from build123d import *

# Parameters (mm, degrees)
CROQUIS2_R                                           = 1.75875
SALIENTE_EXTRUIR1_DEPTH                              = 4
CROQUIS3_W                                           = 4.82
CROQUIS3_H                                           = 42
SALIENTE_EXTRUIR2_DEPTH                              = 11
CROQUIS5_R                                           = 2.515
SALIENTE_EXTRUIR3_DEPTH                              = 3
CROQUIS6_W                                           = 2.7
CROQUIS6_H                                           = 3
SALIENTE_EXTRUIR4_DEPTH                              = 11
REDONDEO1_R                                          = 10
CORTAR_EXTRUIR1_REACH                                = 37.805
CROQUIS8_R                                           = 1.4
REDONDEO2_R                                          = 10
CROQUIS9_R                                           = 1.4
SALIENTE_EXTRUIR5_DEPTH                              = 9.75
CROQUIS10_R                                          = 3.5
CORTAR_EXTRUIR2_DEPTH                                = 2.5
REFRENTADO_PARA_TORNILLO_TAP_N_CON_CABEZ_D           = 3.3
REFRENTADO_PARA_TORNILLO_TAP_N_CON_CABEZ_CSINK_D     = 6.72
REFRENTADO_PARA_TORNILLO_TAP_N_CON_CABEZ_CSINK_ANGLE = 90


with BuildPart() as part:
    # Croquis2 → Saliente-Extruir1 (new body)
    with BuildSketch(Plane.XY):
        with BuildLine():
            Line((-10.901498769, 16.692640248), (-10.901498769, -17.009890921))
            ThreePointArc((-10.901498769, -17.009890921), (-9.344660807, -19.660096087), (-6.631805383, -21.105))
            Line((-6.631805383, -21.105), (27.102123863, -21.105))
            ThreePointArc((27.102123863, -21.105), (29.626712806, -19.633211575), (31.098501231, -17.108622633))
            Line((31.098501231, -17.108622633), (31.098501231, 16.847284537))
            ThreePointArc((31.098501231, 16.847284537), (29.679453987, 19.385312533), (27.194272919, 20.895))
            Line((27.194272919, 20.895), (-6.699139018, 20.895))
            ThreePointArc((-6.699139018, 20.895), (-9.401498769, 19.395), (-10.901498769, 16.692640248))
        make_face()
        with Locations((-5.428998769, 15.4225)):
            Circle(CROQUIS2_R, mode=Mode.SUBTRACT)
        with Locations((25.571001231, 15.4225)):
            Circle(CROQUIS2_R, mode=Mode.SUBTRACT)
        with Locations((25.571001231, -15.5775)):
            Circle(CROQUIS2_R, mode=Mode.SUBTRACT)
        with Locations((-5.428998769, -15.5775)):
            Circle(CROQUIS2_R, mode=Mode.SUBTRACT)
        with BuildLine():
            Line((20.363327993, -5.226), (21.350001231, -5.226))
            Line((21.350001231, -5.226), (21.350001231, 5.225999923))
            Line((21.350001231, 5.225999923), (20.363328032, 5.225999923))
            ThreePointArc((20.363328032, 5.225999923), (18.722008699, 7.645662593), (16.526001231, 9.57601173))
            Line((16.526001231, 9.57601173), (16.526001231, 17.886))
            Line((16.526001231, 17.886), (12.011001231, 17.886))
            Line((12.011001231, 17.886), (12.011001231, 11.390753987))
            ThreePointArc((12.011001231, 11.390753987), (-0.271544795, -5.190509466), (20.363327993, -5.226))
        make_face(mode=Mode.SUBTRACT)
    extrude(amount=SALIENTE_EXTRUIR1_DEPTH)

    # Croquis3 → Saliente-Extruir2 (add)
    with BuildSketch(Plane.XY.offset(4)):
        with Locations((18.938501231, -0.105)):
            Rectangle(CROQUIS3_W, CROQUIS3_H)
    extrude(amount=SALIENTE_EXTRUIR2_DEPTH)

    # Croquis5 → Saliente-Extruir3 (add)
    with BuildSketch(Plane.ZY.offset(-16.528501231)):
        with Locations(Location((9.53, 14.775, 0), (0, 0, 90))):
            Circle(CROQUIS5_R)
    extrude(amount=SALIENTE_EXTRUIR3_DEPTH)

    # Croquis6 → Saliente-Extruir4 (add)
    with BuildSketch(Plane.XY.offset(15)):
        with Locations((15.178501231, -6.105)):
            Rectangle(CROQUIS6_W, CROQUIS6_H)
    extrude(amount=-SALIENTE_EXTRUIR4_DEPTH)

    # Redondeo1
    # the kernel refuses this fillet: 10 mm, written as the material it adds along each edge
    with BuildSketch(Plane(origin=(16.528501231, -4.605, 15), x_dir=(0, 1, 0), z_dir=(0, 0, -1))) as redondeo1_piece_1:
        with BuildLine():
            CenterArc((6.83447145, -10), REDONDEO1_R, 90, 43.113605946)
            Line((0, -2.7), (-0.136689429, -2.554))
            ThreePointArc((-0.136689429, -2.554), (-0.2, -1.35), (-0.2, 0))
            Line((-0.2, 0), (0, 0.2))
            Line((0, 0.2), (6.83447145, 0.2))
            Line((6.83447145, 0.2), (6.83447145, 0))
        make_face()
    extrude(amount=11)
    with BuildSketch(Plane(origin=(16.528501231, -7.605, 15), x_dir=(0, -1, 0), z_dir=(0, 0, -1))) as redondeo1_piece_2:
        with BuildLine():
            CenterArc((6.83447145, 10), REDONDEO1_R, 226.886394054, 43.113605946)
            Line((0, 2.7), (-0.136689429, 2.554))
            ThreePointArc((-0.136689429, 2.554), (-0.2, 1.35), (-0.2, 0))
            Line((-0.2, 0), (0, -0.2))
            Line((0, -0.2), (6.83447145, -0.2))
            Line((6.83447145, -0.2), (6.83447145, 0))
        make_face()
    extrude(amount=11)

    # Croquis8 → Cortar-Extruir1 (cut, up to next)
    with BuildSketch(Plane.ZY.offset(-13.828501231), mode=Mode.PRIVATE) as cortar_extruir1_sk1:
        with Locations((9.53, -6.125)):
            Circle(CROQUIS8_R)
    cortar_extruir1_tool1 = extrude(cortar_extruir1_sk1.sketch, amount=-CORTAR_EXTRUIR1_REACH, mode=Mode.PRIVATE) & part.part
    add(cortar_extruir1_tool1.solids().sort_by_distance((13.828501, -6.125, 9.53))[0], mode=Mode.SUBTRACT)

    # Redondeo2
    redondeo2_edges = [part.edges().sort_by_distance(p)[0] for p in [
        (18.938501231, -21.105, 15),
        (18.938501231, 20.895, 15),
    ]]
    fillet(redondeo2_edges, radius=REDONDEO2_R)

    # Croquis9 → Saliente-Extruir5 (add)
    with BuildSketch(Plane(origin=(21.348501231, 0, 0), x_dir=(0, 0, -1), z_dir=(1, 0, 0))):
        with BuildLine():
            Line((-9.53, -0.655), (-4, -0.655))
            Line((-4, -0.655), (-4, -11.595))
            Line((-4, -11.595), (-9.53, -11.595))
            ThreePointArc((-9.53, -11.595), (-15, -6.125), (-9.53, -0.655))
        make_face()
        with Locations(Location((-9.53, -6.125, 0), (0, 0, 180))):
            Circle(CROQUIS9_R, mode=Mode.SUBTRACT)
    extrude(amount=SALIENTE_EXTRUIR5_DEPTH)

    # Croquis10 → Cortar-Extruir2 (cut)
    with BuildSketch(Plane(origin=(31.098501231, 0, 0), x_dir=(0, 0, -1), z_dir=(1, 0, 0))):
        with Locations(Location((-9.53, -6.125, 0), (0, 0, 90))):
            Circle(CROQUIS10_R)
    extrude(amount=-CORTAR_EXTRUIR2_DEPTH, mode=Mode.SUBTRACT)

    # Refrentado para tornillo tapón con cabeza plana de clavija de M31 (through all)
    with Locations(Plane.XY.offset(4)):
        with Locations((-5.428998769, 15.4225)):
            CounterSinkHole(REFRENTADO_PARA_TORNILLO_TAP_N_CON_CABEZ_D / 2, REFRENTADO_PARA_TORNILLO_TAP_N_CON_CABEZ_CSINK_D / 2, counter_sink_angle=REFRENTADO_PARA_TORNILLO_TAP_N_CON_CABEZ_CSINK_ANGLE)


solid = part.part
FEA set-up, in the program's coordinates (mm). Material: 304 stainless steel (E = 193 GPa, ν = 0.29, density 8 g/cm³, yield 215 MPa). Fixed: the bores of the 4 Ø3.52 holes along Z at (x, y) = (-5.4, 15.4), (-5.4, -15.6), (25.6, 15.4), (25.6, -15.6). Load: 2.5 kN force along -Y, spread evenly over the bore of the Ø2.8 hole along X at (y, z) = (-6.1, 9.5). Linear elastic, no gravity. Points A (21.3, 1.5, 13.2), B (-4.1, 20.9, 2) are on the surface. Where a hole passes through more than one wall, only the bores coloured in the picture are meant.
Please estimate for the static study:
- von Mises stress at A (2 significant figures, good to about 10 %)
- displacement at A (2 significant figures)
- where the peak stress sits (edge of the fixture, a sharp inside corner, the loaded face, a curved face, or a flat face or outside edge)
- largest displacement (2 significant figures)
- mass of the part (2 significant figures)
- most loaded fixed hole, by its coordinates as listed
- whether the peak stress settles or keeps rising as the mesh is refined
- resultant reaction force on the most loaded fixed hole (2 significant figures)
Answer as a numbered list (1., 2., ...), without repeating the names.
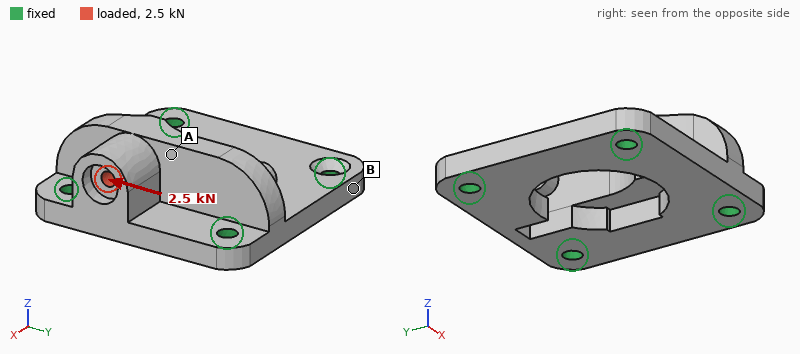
1. 22 MPa
2. 4.0 µm
3. a sharp inside corner
4. 6.2 µm
5. 65 g
6. (25.6, -15.6)
7. keeps rising
8. 1.5 kN
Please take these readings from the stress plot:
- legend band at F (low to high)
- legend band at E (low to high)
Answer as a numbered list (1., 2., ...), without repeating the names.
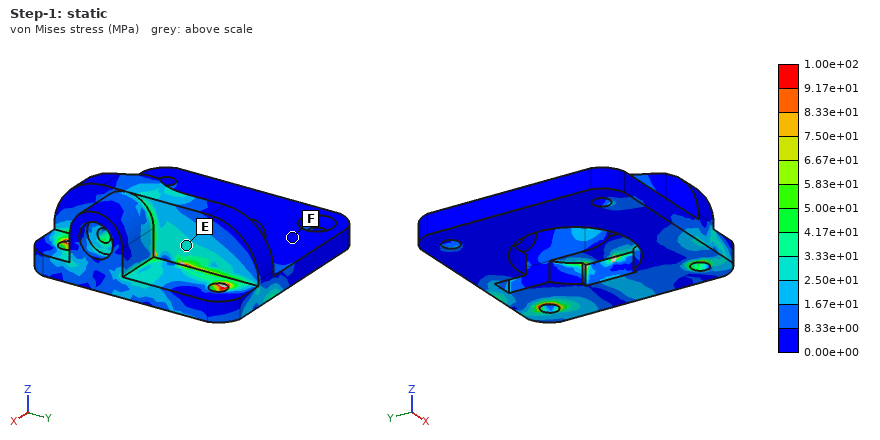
1. 0.00e+00 to 8.33e+00 MPa
2. 2.50e+01 to 3.33e+01 MPa
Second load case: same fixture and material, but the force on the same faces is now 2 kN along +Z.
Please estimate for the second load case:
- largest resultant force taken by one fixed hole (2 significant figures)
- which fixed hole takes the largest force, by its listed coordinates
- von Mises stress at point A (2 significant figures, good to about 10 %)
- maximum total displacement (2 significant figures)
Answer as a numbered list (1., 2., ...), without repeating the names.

1. 1.4 kN
2. (25.6, -15.6)
3. 32 MPa
4. 12 µm
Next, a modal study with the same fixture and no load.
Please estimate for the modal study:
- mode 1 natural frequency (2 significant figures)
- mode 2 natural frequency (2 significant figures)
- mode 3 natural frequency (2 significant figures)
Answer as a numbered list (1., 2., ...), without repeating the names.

1. 10 kHz
2. 17 kHz
3. 19 kHz
